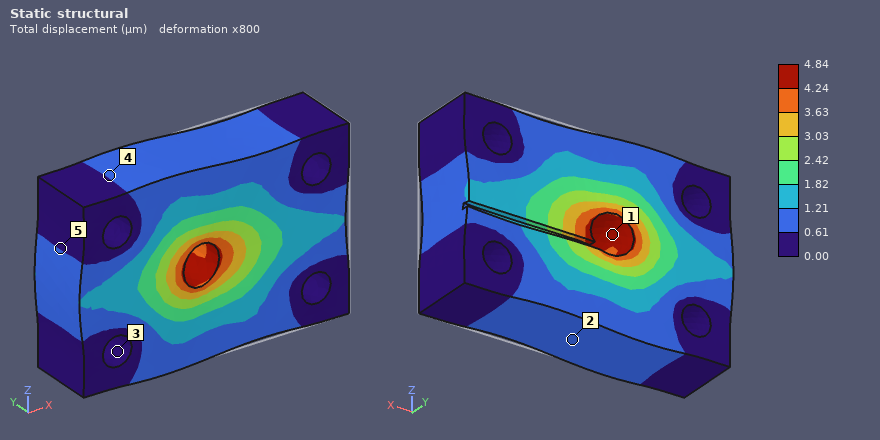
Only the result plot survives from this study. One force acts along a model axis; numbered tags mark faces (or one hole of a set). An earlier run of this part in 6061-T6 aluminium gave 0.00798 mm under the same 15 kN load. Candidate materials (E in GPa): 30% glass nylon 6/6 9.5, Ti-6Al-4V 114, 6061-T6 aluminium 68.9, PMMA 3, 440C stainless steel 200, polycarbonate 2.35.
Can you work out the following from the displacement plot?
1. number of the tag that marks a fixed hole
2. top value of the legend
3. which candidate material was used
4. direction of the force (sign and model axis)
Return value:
3
4.84 µm
Ti-6Al-4V
-X
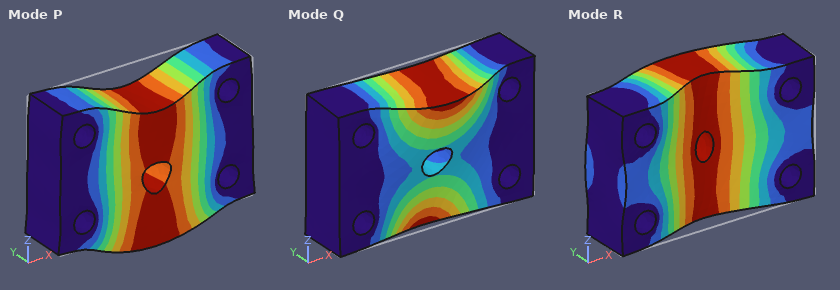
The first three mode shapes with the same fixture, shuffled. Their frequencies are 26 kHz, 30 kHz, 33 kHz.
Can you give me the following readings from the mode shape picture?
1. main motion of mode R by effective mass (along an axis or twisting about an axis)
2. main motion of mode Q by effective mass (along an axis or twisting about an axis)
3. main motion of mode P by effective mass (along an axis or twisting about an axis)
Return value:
along Y
twisting about X
along Z
